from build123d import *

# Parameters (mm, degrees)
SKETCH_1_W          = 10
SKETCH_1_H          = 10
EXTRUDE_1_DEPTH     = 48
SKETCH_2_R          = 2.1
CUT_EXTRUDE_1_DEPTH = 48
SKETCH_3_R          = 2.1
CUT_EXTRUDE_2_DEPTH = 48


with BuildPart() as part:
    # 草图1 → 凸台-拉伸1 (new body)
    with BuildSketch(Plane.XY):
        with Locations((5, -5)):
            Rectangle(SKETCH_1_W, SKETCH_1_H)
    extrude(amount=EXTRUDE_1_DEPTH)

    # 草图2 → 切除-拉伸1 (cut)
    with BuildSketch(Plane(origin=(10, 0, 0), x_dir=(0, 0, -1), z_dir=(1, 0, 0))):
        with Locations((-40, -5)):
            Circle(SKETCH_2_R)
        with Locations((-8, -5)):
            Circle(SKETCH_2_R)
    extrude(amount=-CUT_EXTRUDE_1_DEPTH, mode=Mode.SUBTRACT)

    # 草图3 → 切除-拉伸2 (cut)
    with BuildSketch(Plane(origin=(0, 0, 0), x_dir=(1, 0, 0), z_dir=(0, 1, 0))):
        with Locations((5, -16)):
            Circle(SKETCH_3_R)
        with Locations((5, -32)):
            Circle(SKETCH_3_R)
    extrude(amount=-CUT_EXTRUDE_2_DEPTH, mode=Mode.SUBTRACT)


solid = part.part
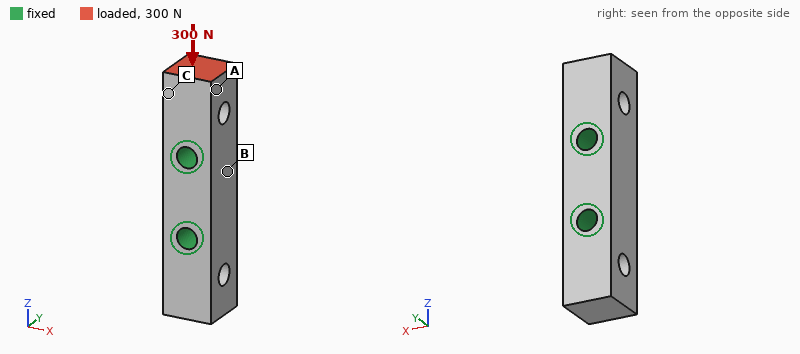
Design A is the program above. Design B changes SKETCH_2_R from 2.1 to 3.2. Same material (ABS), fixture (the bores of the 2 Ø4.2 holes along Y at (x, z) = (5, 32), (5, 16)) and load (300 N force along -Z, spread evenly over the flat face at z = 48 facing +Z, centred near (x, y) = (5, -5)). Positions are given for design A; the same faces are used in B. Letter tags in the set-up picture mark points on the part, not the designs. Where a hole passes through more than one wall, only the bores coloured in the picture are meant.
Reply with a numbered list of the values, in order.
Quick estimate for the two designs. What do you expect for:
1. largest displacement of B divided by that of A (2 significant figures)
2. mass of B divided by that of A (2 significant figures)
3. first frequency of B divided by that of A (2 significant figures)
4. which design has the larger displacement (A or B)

1. 1.6
2. 0.91
3. 0.90
4. B
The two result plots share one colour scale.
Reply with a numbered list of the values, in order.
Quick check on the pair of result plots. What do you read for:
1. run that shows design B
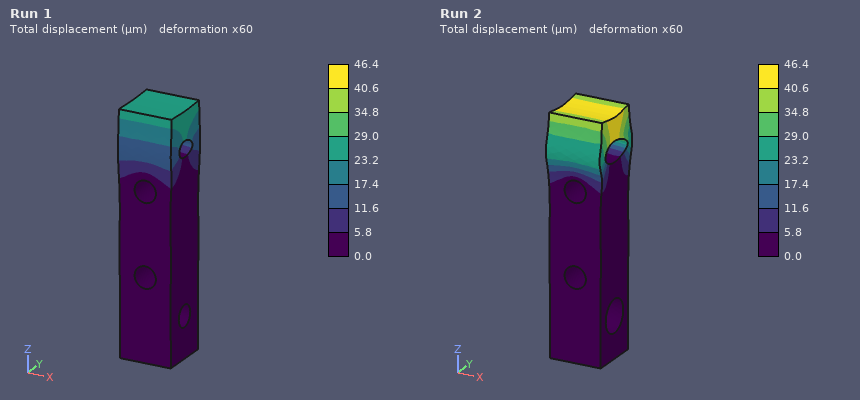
1. Run 2
